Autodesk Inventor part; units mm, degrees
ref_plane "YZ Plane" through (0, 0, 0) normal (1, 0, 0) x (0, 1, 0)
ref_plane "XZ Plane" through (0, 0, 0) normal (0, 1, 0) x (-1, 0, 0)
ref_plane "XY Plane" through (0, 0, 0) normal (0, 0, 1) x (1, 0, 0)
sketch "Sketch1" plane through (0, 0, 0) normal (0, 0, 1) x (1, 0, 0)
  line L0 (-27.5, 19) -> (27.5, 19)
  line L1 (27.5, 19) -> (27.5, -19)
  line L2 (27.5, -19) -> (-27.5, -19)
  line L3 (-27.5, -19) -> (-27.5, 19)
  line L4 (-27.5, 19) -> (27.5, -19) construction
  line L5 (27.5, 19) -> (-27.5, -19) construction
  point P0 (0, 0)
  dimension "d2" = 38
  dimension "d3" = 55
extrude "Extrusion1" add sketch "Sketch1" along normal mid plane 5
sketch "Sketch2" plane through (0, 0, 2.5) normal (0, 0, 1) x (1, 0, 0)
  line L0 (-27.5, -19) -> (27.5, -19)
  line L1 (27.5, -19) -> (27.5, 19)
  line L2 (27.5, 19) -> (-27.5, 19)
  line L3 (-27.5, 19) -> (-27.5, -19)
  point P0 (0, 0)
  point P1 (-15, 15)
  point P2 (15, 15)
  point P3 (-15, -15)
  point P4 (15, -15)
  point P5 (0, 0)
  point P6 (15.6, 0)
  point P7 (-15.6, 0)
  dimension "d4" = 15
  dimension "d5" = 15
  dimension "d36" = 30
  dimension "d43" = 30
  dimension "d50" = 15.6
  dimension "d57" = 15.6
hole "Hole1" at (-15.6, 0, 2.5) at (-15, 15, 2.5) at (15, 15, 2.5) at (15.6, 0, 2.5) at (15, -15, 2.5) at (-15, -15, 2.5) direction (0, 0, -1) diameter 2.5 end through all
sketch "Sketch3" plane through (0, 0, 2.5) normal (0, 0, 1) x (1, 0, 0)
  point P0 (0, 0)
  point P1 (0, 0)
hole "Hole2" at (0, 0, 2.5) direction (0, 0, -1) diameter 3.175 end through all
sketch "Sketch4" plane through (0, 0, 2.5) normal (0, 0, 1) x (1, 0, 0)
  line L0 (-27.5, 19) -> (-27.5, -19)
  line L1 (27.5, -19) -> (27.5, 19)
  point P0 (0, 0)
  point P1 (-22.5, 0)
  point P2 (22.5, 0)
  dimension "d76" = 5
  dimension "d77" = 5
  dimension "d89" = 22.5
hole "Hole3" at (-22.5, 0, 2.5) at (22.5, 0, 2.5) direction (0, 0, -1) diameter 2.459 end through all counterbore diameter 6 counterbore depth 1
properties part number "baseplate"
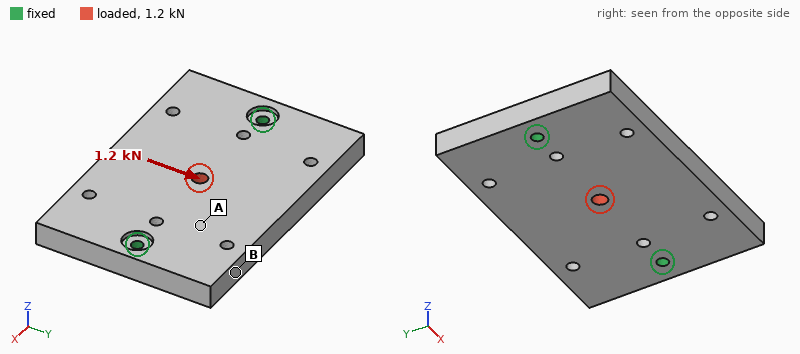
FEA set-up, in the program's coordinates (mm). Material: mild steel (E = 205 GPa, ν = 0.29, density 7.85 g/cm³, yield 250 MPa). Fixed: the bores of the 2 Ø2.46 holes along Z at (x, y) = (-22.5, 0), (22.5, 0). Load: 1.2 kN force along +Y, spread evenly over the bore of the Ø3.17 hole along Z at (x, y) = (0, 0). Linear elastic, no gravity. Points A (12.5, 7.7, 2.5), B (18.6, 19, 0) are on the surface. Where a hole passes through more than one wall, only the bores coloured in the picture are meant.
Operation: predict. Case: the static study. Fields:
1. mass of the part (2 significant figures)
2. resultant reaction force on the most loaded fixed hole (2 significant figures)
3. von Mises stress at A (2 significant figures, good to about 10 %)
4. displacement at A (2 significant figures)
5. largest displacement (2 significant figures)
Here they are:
80 g
600 N
7.4 MPa
1.3 µm
2.3 µm
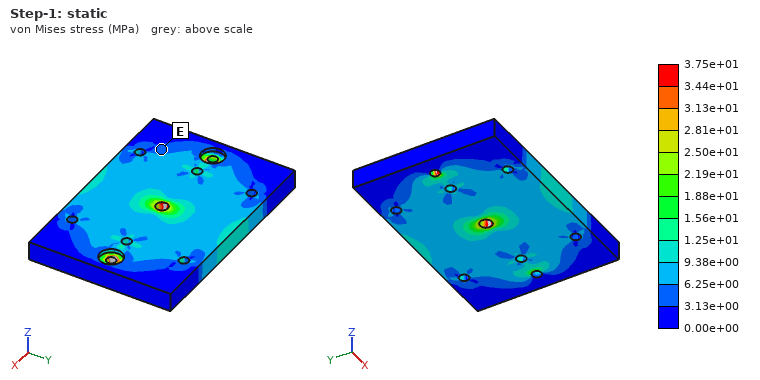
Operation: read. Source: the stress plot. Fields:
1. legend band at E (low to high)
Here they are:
3.13e+00 to 6.25e+00 MPa
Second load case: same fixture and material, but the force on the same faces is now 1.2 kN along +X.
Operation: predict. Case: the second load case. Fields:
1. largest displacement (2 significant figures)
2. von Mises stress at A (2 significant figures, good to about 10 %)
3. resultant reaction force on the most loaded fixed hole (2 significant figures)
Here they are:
1.4 µm
3.8 MPa
600 N
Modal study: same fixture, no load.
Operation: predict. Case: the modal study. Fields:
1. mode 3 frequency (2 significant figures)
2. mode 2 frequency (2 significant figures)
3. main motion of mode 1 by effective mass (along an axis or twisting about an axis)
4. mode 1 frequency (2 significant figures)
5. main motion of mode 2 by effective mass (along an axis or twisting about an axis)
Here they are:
10 kHz
6800 Hz
twisting about X
4900 Hz
along Z
